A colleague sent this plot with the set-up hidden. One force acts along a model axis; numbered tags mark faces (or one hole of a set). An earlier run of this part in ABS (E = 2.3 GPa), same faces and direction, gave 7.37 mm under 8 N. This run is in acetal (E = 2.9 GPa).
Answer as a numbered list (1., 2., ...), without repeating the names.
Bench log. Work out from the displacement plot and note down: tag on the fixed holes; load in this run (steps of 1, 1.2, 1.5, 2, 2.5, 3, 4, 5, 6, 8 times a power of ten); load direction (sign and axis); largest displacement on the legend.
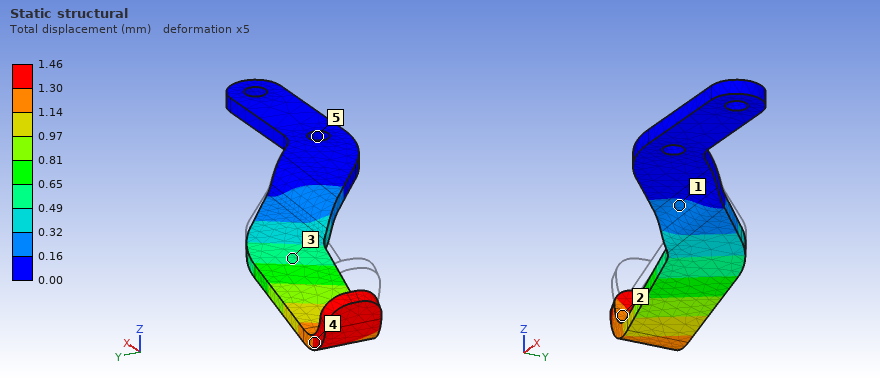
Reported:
1. 5
2. 2 N
3. -Z
4. 1.46 mm
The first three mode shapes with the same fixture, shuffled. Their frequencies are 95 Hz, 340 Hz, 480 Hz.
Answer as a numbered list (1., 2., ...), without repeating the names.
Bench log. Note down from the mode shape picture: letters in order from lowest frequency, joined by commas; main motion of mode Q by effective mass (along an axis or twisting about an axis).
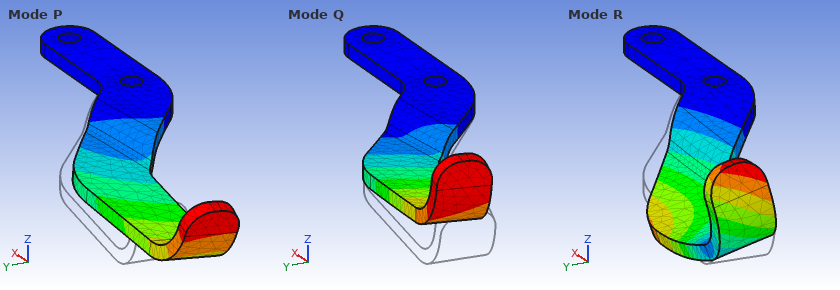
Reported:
1. Q, P, R
2. along Z
